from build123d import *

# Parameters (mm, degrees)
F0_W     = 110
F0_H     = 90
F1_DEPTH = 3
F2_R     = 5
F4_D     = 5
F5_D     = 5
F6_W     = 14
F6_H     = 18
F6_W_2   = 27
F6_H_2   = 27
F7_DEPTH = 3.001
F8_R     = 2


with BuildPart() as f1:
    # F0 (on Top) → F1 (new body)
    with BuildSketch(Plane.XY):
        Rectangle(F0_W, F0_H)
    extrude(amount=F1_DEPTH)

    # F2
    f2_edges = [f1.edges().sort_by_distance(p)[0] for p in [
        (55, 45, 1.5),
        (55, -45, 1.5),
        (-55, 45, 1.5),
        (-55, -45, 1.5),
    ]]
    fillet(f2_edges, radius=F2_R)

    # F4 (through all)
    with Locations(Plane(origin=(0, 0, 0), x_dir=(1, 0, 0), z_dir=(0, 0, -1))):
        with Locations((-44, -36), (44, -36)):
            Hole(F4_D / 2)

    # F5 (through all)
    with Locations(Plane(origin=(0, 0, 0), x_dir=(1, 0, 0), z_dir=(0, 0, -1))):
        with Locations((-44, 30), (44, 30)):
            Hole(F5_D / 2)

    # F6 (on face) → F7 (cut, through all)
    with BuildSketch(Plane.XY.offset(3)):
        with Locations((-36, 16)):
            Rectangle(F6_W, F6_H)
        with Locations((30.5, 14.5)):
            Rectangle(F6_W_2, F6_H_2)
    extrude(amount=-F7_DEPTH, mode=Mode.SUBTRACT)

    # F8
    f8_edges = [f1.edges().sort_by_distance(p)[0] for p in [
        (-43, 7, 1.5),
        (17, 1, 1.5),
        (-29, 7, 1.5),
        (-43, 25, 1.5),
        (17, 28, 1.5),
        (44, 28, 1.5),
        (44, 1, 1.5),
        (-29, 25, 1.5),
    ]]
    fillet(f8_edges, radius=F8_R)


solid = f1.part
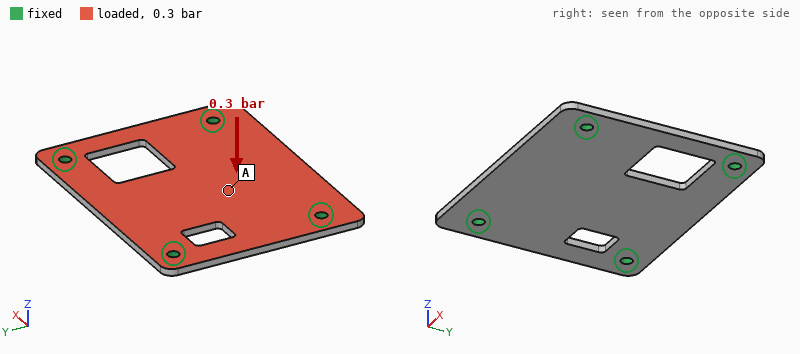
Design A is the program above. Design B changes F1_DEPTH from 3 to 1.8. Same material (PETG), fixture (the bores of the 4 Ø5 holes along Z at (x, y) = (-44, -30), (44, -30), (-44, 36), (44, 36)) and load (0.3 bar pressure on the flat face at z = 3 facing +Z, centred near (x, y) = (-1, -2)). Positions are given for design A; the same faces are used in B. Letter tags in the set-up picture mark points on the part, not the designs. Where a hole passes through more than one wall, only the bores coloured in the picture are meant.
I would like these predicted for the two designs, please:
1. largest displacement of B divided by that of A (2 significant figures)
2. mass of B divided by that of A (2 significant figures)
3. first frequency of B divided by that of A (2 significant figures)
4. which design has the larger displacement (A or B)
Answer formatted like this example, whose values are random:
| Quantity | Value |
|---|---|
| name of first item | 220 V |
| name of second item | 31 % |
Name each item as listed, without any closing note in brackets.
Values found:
| Quantity | Value |
|---|---|
| largest displacement of B divided by that of A | 4.4 |
| mass of B divided by that of A | 0.60 |
| first frequency of B divided by that of A | 0.62 |
| which design has the larger displacement | B |
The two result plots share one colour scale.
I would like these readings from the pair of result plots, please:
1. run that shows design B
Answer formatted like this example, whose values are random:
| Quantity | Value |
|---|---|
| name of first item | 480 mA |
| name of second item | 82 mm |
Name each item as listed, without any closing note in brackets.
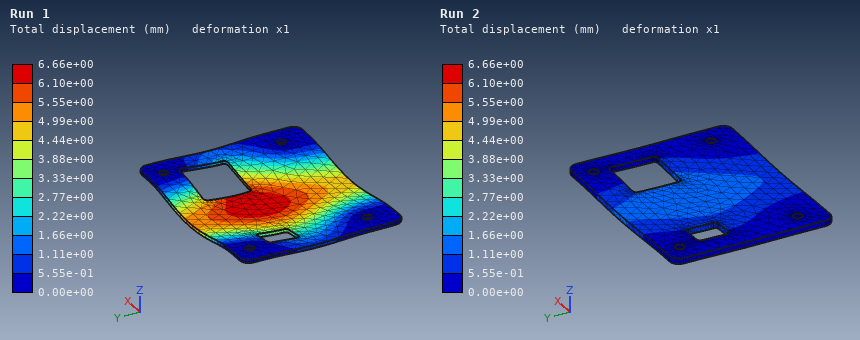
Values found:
| Quantity | Value |
|---|---|
| run that shows design B | Run 1 |
